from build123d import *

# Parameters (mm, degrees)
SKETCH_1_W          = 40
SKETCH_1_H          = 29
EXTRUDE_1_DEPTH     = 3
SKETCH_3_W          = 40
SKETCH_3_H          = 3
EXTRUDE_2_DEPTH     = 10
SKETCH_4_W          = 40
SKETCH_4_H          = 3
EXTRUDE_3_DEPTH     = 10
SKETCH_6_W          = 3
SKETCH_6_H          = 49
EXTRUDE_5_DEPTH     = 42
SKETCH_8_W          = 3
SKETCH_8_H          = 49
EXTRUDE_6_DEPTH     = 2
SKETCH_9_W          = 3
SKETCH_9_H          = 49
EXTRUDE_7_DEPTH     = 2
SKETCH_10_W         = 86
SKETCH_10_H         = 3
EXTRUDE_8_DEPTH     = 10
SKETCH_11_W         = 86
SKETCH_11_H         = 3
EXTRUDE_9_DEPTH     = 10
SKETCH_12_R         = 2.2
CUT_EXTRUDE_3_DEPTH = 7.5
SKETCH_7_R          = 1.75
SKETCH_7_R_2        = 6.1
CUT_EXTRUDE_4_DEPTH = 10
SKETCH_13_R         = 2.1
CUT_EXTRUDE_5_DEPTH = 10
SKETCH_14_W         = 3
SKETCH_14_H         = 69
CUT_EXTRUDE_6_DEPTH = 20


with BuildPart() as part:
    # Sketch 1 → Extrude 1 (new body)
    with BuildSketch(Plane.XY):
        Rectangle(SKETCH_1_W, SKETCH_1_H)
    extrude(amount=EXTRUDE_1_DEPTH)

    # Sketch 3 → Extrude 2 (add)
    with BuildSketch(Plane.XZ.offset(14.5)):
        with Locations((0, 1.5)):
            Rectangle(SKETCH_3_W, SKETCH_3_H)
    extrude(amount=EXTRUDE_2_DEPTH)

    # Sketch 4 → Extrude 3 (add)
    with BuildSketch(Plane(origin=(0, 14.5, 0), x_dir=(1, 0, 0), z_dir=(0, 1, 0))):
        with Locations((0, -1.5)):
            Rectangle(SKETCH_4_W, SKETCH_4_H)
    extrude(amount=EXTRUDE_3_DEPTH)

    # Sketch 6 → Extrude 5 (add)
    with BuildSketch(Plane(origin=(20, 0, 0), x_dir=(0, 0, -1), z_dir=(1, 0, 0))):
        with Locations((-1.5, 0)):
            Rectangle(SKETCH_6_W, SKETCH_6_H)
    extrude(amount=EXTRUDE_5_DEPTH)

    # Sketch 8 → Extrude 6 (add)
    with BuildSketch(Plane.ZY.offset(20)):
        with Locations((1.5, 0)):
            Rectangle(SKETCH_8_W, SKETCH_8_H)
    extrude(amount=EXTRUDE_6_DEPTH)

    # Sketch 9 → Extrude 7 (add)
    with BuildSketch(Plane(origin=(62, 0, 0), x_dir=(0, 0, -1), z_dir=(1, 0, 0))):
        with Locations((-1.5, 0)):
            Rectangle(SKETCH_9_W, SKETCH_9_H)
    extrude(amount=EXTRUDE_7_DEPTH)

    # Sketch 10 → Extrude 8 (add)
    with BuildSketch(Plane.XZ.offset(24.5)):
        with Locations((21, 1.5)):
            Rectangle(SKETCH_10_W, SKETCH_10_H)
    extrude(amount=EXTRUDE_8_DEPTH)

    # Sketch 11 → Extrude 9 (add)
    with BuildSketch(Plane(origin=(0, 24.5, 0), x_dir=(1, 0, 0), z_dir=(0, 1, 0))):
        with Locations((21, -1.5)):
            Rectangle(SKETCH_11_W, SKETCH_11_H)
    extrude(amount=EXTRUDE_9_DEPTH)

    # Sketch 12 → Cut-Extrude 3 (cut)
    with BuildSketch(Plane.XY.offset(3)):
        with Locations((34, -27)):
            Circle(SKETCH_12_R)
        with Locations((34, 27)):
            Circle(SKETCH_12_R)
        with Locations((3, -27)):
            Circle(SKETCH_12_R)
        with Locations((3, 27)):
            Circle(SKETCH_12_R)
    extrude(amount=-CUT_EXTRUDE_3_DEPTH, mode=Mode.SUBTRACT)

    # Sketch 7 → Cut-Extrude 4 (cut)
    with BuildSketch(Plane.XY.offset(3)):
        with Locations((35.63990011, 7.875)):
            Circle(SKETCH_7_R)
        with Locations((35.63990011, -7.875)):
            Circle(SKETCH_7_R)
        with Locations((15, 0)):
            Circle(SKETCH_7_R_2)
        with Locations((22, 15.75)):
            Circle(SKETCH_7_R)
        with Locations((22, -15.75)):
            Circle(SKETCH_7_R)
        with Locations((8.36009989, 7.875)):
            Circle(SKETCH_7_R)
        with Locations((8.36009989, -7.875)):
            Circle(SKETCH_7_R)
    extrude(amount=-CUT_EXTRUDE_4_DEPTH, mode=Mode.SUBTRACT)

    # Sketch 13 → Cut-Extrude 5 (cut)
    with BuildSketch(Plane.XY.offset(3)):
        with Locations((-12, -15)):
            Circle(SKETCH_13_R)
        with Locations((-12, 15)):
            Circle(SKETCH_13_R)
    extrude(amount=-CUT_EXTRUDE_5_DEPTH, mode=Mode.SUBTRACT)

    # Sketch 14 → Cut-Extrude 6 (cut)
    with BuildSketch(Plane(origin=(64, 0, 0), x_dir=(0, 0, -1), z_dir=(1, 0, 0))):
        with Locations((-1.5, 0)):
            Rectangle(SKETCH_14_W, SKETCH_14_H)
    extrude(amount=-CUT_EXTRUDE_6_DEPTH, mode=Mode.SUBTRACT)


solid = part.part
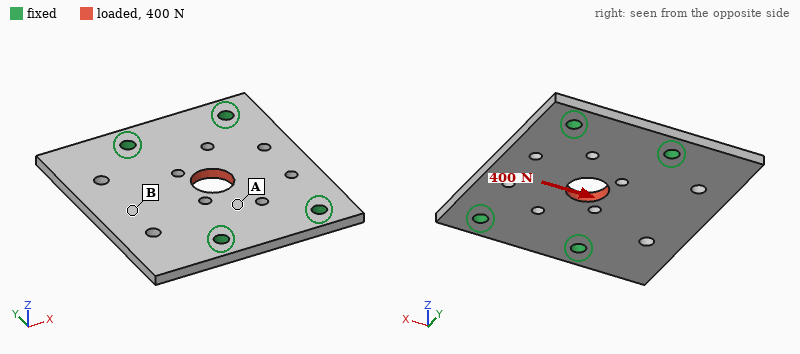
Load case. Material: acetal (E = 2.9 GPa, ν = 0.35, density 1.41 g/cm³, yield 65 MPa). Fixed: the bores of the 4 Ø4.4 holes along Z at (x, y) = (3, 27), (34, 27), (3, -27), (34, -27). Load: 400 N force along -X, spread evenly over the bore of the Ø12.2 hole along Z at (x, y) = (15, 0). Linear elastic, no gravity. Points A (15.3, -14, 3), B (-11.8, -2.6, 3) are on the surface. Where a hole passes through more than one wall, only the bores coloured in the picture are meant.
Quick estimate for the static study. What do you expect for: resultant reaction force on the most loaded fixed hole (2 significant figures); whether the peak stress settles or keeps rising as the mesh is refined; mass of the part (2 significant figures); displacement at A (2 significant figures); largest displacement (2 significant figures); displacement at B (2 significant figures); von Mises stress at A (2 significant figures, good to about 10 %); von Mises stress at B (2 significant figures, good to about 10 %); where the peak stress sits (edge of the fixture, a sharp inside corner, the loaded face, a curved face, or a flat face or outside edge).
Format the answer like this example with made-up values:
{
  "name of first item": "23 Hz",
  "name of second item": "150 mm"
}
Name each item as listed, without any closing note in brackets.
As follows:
{
  "resultant reaction force on the most loaded fixed hole": "120 N",
  "whether the peak stress settles or keeps rising as the mesh is refined": "keeps rising",
  "mass of the part": "18 g",
  "displacement at A": "20 µm",
  "largest displacement": "41 µm",
  "displacement at B": "25 µm",
  "von Mises stress at A": "2.6 MPa",
  "von Mises stress at B": "1.2 MPa",
  "where the peak stress sits": "edge of the fixture"
}
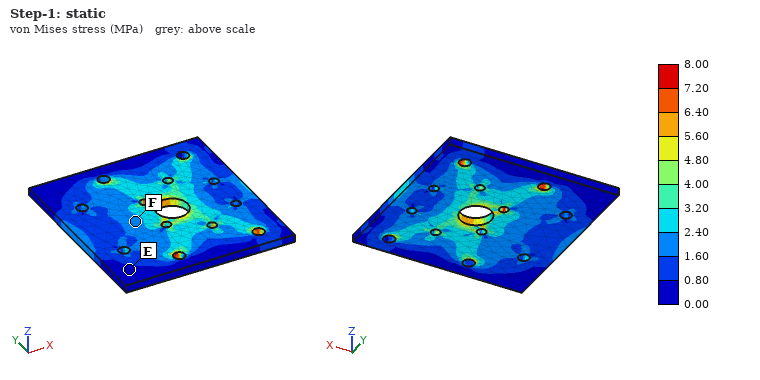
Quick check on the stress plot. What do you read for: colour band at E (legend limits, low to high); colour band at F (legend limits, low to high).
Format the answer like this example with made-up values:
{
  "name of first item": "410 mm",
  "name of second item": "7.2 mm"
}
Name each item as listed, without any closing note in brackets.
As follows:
{
  "colour band at E": "0.00 to 0.80 MPa",
  "colour band at F": "1.60 to 2.40 MPa"
}
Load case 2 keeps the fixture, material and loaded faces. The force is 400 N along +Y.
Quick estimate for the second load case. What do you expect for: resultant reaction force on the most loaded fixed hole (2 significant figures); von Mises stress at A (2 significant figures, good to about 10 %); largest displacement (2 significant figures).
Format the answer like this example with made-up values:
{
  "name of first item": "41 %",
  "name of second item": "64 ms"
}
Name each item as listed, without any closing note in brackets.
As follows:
{
  "resultant reaction force on the most loaded fixed hole": "120 N",
  "von Mises stress at A": "2.5 MPa",
  "largest displacement": "28 µm"
}
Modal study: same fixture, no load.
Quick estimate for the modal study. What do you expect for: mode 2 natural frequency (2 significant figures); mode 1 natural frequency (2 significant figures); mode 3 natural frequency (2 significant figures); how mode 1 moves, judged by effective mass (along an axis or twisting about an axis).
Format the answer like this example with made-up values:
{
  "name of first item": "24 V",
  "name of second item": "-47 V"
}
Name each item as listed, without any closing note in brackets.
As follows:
{
  "mode 2 natural frequency": "1500 Hz",
  "mode 1 natural frequency": "870 Hz",
  "mode 3 natural frequency": "1500 Hz",
  "how mode 1 moves, judged by effective mass": "along Z"
}
